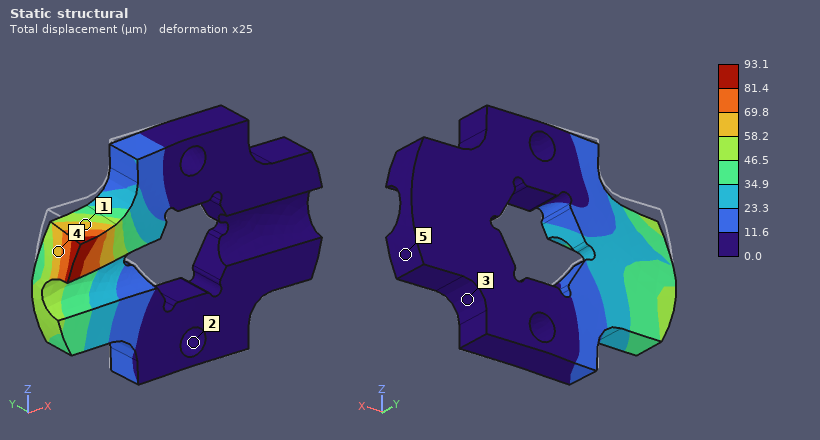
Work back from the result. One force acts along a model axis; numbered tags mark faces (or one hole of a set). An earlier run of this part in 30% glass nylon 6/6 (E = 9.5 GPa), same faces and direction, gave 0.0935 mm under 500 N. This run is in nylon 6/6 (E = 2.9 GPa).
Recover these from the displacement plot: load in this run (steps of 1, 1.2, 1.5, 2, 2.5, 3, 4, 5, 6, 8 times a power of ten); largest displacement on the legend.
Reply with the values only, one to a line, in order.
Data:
150 N
93.1 µm
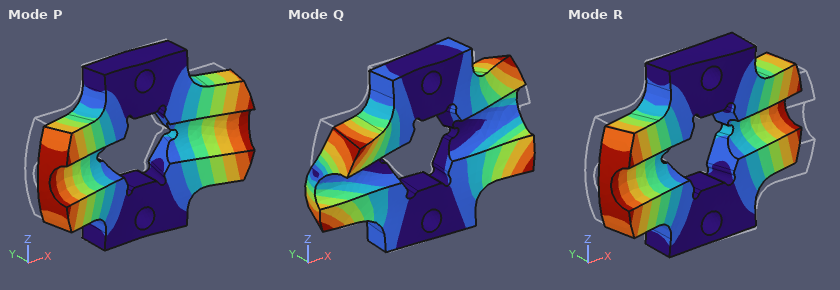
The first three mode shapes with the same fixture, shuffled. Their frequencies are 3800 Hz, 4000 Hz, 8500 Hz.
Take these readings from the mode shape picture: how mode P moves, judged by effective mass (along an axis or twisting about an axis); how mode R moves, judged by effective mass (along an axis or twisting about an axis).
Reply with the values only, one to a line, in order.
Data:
along Y
twisting about Z
